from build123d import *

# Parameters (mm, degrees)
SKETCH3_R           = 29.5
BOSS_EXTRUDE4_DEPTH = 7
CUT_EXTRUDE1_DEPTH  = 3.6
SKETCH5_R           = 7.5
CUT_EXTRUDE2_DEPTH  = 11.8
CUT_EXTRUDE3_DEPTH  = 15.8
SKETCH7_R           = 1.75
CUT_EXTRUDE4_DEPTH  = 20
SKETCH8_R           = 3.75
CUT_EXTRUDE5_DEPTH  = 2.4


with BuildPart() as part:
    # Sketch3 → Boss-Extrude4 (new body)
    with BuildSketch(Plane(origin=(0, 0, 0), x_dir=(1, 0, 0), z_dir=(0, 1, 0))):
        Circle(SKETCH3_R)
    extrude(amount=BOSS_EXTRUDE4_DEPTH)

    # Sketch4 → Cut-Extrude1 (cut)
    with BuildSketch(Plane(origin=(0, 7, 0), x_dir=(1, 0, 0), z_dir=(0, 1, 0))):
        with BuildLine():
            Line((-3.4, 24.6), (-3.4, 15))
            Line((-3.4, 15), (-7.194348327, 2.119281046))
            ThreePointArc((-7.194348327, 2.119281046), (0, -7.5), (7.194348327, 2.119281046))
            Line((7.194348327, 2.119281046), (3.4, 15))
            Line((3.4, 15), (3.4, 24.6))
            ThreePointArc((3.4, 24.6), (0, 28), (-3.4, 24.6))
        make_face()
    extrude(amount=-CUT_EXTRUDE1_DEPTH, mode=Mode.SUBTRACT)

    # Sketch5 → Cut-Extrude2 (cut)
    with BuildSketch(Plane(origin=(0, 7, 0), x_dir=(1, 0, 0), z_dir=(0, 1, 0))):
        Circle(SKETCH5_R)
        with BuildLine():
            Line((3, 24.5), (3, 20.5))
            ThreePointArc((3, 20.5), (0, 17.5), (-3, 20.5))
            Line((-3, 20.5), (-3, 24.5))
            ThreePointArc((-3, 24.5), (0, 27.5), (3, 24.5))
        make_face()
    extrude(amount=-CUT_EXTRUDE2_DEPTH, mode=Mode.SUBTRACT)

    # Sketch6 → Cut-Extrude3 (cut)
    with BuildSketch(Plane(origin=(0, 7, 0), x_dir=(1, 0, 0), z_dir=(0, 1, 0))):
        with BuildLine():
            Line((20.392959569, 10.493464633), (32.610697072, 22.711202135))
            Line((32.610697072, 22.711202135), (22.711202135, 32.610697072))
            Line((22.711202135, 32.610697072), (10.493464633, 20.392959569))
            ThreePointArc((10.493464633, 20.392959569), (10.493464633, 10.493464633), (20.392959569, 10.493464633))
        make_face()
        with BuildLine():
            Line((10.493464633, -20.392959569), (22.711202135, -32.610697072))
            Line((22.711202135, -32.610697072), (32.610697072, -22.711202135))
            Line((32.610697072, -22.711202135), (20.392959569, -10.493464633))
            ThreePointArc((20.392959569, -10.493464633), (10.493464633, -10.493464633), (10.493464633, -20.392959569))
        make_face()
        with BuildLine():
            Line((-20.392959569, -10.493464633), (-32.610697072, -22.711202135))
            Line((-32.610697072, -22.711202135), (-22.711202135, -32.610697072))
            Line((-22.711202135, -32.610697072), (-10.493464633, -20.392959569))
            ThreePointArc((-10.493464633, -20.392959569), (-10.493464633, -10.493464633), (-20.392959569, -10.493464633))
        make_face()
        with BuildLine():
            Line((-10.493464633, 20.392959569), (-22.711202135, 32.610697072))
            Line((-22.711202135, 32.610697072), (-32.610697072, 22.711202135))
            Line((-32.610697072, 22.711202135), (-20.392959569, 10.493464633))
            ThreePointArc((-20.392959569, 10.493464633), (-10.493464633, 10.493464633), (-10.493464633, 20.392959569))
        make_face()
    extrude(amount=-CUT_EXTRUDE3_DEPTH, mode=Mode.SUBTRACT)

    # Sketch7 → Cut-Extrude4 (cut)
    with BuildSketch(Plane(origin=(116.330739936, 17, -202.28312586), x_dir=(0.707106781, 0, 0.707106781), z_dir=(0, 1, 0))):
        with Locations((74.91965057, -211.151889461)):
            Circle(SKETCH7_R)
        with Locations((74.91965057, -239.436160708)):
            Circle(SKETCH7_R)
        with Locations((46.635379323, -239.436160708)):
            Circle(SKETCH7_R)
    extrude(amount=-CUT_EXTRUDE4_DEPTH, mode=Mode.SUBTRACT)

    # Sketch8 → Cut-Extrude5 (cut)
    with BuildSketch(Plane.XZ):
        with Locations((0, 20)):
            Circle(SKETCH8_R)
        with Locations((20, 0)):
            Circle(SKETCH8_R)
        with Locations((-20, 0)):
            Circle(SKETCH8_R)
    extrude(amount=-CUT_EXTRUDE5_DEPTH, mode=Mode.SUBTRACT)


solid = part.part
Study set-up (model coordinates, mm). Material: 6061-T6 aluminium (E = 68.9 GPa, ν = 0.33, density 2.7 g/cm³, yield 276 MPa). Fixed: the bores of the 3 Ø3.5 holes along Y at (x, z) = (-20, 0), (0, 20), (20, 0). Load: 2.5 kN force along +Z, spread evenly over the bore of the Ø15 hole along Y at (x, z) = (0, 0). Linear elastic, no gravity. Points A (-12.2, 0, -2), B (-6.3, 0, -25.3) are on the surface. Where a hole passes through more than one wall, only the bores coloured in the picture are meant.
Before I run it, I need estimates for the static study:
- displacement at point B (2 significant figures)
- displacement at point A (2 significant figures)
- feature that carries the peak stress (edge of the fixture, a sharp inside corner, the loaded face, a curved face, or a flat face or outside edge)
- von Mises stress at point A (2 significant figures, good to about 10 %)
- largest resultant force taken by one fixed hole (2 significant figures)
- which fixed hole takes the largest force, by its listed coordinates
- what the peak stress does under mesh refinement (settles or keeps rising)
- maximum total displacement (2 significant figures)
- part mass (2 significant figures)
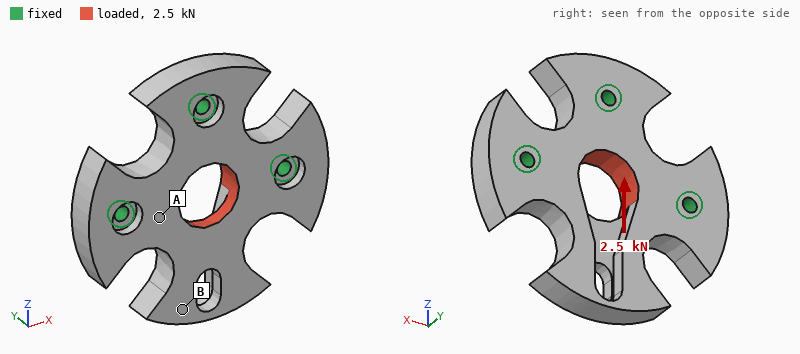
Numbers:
18 µm
5.3 µm
edge of the fixture
12 MPa
1.5 kN
(0, 20)
keeps rising
21 µm
31 g
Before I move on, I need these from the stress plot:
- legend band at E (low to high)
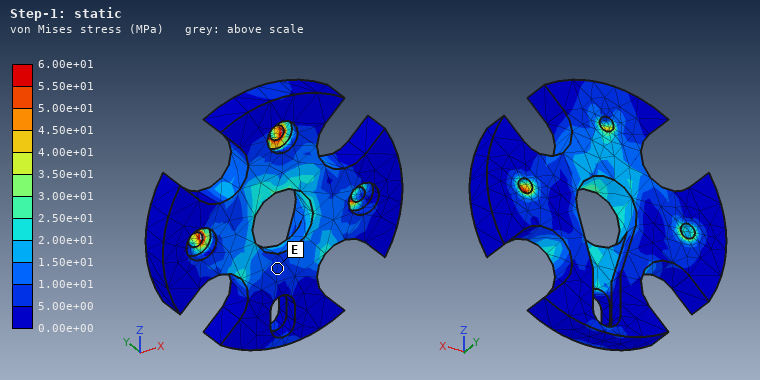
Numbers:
5.00e+00 to 1.00e+01 MPa
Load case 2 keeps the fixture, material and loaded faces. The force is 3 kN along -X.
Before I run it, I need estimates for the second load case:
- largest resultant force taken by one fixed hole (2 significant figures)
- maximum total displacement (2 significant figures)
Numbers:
1.3 kN
5.8 µm
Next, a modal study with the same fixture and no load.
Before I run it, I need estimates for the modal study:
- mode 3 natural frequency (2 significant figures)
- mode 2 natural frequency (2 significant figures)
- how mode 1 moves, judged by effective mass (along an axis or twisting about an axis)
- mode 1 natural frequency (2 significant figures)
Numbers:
13 kHz
9900 Hz
along Y
4500 Hz
